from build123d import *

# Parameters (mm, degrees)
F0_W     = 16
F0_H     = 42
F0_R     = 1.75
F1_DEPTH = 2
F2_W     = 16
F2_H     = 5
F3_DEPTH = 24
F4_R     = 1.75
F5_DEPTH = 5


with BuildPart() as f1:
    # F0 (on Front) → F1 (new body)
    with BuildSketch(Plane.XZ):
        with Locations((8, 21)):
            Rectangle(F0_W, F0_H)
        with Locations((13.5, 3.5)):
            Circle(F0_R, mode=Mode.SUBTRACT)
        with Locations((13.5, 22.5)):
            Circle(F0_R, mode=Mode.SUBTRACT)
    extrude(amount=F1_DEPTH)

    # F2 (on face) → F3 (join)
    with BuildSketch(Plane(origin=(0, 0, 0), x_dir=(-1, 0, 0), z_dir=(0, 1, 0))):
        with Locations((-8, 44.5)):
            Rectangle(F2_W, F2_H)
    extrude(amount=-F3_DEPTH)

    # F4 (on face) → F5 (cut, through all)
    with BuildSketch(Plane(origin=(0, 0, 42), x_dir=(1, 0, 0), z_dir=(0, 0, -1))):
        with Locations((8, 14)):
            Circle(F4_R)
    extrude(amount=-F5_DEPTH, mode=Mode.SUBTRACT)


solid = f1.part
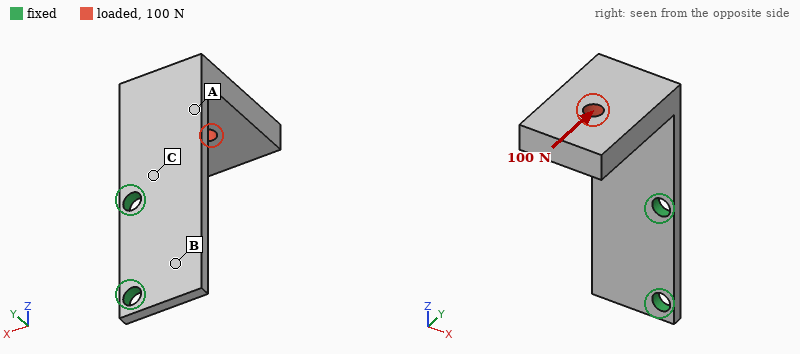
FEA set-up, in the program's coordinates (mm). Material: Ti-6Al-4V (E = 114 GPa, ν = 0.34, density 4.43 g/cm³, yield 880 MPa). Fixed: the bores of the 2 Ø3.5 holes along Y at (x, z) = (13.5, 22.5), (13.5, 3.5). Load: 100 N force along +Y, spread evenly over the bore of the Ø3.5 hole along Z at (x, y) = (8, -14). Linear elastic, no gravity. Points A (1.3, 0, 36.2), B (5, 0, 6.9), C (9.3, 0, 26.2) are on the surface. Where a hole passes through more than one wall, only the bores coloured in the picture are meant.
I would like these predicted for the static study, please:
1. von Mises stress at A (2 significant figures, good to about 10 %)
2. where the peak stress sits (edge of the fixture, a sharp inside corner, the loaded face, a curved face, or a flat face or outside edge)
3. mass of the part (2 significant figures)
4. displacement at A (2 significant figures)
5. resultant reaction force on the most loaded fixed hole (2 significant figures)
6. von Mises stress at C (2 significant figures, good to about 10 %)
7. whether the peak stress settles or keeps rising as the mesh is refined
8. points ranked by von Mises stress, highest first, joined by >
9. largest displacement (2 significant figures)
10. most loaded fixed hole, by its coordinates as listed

76 MPa
edge of the fixture
14 g
0.17 mm
130 N
160 MPa
keeps rising
C > A > B
0.60 mm
(13.5, 22.5)
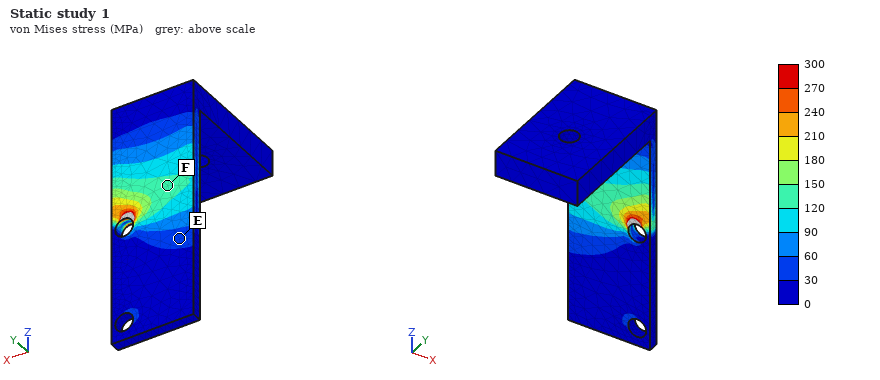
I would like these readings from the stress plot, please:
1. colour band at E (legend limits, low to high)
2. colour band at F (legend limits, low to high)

30 to 60 MPa
120 to 150 MPa
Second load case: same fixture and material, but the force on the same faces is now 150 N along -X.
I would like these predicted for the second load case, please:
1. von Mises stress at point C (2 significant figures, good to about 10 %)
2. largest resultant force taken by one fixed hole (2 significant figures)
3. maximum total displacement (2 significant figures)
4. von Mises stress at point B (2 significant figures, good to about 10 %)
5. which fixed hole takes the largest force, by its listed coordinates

120 MPa
310 N
0.54 mm
27 MPa
(13.5, 22.5)
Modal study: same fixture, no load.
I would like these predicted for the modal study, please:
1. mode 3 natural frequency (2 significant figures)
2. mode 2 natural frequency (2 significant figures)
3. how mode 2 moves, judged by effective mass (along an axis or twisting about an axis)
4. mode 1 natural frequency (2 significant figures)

2900 Hz
1200 Hz
along X
730 Hz
